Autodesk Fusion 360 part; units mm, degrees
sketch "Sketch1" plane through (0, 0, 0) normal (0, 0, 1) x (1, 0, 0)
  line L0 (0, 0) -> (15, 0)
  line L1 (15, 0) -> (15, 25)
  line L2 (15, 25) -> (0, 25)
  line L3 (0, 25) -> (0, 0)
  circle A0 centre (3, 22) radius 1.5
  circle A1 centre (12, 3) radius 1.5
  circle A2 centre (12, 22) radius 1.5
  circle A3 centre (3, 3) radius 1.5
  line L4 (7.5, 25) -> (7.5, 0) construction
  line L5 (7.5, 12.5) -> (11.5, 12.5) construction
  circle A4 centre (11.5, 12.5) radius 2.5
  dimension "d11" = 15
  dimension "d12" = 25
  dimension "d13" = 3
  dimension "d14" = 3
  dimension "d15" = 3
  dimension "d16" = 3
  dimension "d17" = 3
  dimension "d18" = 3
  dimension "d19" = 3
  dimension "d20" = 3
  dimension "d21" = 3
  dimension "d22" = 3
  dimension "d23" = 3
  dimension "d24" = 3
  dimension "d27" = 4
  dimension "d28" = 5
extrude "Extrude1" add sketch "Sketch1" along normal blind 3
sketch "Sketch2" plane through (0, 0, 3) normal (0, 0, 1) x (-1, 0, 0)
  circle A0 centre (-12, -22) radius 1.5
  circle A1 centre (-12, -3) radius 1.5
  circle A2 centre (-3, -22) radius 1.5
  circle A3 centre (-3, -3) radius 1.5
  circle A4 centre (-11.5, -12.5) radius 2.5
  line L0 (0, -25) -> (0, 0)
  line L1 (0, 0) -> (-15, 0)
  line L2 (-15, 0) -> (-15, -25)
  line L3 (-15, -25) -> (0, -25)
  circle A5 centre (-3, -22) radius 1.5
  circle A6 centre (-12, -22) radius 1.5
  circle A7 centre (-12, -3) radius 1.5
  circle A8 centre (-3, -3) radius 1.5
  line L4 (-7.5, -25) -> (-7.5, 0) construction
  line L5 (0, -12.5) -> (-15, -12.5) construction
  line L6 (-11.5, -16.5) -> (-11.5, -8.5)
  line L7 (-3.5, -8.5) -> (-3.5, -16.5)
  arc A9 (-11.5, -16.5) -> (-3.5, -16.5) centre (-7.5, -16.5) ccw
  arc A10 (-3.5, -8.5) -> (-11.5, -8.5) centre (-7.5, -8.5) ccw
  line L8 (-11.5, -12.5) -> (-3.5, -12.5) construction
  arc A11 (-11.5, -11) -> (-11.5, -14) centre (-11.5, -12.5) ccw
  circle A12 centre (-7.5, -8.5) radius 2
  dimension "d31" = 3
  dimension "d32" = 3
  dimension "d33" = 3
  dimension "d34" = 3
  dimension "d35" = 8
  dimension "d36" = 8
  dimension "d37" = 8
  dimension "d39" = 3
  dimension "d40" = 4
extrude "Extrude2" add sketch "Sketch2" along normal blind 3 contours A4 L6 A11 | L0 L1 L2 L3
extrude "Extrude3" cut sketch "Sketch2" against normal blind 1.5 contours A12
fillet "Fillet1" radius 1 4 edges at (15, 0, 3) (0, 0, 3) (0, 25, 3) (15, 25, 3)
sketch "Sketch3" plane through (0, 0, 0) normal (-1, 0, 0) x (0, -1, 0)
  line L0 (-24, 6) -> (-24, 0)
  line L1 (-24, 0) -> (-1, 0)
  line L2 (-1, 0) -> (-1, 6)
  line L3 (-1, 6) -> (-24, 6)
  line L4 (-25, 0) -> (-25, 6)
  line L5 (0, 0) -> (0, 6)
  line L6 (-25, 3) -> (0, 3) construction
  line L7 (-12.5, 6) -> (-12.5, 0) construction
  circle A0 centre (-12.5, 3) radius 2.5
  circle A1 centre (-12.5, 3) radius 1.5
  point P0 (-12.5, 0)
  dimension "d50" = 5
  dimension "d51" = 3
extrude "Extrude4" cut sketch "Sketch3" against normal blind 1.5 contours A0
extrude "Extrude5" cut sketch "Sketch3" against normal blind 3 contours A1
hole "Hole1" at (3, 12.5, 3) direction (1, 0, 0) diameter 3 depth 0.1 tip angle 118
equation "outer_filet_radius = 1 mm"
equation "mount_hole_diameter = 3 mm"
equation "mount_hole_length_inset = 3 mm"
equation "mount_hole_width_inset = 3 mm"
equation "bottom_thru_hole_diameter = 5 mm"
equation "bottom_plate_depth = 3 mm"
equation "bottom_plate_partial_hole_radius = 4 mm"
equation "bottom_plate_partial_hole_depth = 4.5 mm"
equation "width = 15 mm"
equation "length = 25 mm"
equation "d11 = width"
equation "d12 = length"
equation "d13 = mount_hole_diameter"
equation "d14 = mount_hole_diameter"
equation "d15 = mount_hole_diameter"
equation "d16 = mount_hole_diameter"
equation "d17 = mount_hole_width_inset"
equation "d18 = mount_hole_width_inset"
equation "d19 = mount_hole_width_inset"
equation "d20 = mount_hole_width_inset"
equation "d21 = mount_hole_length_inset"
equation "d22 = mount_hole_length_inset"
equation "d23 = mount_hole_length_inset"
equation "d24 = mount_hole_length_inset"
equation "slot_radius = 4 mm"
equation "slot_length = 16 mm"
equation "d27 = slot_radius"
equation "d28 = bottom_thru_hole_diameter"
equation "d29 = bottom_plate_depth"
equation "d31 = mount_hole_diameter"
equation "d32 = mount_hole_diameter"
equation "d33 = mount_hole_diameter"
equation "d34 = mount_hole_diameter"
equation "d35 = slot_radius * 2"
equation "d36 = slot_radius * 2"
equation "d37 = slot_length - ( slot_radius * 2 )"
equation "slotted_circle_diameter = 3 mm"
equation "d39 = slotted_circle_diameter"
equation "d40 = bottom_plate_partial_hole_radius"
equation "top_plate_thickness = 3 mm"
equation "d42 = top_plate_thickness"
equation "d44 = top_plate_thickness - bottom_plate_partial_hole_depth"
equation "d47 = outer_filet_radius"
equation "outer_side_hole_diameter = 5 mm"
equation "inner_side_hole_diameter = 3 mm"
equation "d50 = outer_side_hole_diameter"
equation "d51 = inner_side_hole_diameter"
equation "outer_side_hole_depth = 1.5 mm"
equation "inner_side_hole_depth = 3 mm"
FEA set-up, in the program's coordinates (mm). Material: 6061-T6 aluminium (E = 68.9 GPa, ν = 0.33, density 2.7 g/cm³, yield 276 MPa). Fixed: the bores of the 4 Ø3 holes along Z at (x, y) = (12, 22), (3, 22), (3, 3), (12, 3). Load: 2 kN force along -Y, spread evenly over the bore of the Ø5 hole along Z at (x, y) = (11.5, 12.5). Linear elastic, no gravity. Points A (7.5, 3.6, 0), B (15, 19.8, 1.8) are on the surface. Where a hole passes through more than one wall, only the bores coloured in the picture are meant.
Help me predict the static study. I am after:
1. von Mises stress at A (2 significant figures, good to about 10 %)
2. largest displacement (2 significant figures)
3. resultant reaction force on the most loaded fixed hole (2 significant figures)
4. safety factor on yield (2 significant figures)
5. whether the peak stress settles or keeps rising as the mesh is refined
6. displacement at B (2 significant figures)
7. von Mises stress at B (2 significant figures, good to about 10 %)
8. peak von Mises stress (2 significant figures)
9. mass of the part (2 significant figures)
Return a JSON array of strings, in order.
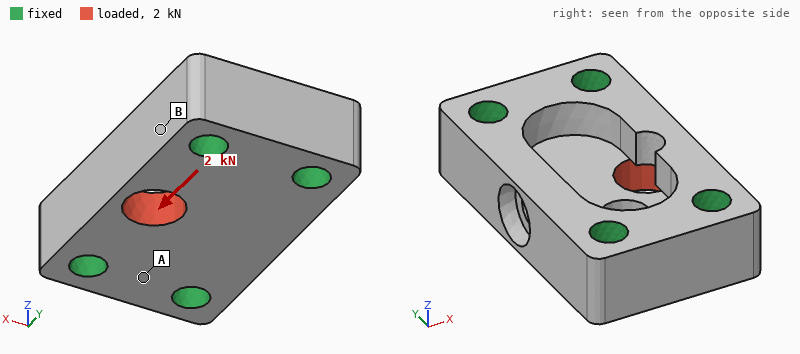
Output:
["9.4 MPa", "4.8 µm", "800 N", "3.3", "settles", "1.1 µm", "22 MPa", "83 MPa", "4.3 g"]
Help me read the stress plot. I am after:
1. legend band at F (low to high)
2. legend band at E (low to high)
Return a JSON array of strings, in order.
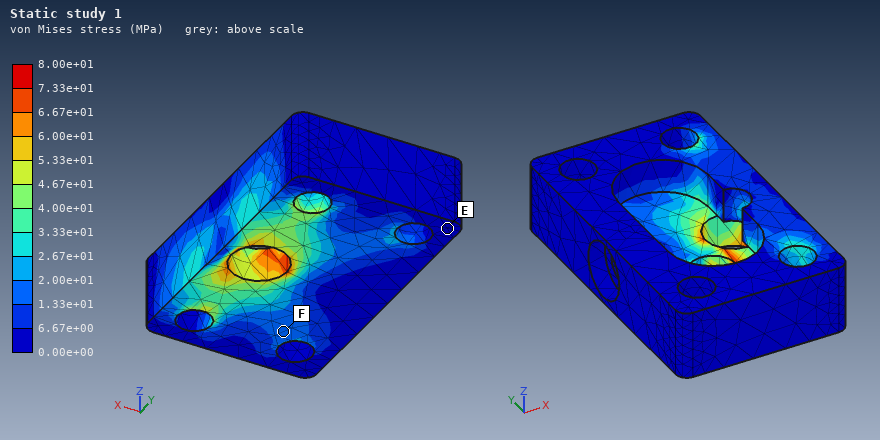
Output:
["1.33e+01 to 2.00e+01 MPa", "0.00e+00 to 6.67e+00 MPa"]
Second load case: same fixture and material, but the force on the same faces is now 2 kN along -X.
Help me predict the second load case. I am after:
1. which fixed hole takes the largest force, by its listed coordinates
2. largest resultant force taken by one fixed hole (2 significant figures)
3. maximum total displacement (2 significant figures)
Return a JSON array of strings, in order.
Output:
["(3, 22)", "680 N", "20 µm"]
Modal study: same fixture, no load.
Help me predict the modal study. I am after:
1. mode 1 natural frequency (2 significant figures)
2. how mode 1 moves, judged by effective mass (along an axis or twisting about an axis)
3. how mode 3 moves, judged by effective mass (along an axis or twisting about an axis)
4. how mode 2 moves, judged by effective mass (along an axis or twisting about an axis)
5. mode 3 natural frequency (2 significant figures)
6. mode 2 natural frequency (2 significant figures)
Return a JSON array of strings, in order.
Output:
["65 kHz", "along Z", "along X", "along X", "80 kHz", "73 kHz"]
